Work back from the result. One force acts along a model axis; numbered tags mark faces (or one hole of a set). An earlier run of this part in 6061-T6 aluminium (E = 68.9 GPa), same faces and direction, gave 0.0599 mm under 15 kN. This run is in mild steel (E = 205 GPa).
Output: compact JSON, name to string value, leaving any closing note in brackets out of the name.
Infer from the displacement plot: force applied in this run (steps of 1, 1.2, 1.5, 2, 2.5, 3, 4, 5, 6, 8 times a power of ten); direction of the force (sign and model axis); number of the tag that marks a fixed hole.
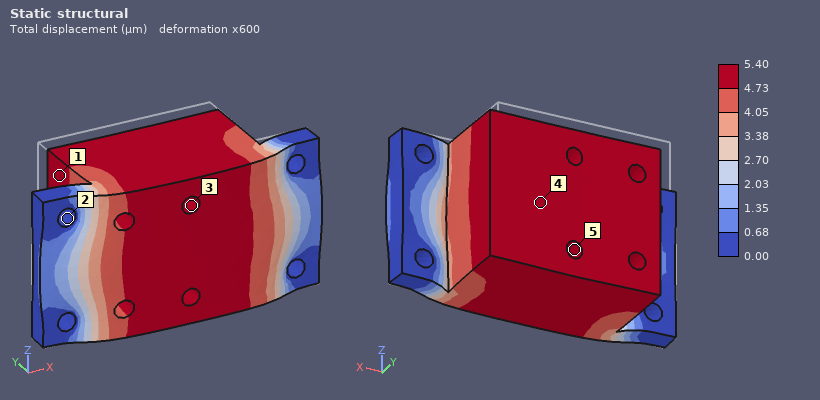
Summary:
{"force applied in this run": "4 kN", "direction of the force": "-Y", "number of the tag that marks a fixed hole": "2"}
